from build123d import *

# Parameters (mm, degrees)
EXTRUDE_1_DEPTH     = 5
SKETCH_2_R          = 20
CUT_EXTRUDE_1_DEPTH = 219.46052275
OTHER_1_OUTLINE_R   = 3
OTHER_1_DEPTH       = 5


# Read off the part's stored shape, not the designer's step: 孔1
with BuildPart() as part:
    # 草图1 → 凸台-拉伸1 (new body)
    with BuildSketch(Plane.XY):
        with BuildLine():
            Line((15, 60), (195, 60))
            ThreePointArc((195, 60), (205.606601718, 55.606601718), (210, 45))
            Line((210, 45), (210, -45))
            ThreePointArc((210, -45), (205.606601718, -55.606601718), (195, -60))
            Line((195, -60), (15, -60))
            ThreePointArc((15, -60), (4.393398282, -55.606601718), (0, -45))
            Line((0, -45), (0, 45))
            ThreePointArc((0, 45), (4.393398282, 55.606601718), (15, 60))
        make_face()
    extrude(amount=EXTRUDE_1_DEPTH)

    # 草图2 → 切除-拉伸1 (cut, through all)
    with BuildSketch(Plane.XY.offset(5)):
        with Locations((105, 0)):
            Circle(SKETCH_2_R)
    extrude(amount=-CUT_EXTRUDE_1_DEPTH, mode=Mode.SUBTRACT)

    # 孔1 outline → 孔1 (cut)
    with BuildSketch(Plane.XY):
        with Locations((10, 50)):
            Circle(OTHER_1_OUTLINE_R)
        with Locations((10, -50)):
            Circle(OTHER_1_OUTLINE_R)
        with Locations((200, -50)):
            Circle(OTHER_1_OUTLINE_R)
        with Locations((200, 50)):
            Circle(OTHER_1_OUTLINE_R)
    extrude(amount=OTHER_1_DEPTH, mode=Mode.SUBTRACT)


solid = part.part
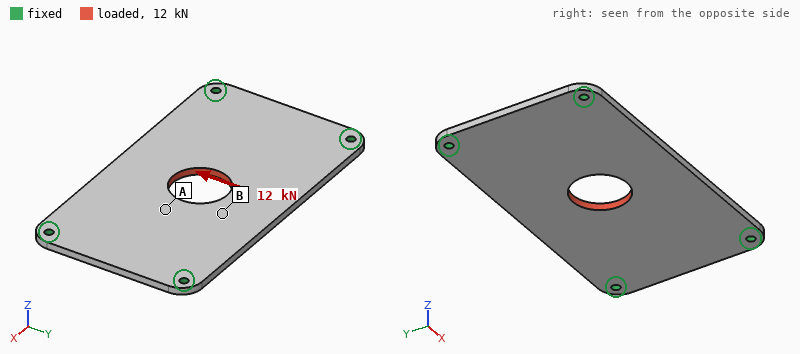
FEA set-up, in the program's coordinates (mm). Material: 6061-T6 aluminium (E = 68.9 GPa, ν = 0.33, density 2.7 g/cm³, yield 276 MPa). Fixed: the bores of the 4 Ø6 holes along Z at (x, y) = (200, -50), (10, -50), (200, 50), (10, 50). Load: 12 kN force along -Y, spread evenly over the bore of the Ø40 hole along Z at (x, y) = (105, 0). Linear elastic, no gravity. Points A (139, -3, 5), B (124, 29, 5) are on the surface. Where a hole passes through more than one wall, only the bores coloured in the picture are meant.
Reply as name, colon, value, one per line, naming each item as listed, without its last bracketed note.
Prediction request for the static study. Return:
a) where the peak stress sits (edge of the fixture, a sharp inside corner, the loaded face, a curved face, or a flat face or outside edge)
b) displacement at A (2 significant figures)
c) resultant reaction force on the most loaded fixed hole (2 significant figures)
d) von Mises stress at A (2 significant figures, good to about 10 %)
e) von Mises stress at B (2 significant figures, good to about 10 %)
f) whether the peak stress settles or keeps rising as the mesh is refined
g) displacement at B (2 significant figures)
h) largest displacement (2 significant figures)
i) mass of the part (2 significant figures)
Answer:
where the peak stress sits: edge of the fixture
displacement at A: 40 µm
resultant reaction force on the most loaded fixed hole: 4.0 kN
von Mises stress at A: 26 MPa
von Mises stress at B: 18 MPa
whether the peak stress settles or keeps rising as the mesh is refined: keeps rising
displacement at B: 48 µm
largest displacement: 56 µm
mass of the part: 320 g
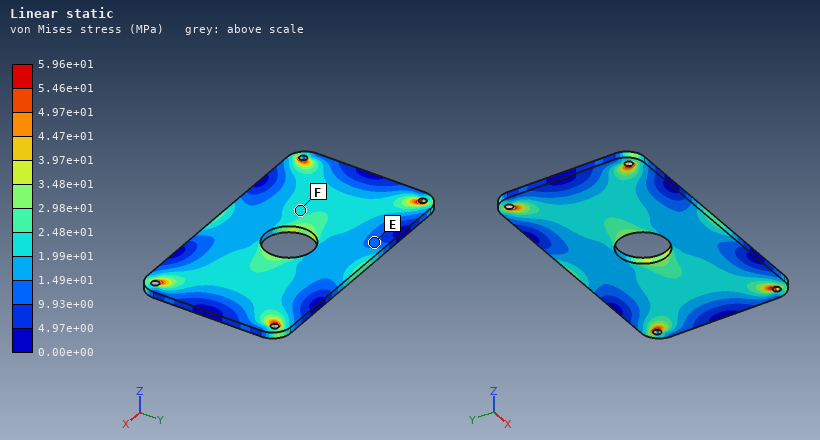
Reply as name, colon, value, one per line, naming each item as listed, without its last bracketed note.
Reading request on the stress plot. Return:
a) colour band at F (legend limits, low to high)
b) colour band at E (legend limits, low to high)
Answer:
colour band at F: 1.99e+01 to 2.48e+01 MPa
colour band at E: 9.93e+00 to 1.49e+01 MPa
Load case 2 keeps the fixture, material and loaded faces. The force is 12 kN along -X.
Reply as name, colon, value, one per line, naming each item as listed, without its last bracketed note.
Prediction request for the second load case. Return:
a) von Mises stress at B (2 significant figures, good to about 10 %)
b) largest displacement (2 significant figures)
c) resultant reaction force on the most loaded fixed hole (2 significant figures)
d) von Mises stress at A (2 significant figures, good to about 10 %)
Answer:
von Mises stress at B: 13 MPa
largest displacement: 25 µm
resultant reaction force on the most loaded fixed hole: 3.1 kN
von Mises stress at A: 16 MPa
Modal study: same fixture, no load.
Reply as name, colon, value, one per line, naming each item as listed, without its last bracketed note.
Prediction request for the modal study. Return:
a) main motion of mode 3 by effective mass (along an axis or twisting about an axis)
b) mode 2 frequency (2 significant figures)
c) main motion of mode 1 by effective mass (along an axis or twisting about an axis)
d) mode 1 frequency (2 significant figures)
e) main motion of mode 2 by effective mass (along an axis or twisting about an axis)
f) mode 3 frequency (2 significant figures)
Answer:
main motion of mode 3 by effective mass: twisting about Y
mode 2 frequency: 1000 Hz
main motion of mode 1 by effective mass: along Z
mode 1 frequency: 610 Hz
main motion of mode 2 by effective mass: twisting about X
mode 3 frequency: 1600 Hz
